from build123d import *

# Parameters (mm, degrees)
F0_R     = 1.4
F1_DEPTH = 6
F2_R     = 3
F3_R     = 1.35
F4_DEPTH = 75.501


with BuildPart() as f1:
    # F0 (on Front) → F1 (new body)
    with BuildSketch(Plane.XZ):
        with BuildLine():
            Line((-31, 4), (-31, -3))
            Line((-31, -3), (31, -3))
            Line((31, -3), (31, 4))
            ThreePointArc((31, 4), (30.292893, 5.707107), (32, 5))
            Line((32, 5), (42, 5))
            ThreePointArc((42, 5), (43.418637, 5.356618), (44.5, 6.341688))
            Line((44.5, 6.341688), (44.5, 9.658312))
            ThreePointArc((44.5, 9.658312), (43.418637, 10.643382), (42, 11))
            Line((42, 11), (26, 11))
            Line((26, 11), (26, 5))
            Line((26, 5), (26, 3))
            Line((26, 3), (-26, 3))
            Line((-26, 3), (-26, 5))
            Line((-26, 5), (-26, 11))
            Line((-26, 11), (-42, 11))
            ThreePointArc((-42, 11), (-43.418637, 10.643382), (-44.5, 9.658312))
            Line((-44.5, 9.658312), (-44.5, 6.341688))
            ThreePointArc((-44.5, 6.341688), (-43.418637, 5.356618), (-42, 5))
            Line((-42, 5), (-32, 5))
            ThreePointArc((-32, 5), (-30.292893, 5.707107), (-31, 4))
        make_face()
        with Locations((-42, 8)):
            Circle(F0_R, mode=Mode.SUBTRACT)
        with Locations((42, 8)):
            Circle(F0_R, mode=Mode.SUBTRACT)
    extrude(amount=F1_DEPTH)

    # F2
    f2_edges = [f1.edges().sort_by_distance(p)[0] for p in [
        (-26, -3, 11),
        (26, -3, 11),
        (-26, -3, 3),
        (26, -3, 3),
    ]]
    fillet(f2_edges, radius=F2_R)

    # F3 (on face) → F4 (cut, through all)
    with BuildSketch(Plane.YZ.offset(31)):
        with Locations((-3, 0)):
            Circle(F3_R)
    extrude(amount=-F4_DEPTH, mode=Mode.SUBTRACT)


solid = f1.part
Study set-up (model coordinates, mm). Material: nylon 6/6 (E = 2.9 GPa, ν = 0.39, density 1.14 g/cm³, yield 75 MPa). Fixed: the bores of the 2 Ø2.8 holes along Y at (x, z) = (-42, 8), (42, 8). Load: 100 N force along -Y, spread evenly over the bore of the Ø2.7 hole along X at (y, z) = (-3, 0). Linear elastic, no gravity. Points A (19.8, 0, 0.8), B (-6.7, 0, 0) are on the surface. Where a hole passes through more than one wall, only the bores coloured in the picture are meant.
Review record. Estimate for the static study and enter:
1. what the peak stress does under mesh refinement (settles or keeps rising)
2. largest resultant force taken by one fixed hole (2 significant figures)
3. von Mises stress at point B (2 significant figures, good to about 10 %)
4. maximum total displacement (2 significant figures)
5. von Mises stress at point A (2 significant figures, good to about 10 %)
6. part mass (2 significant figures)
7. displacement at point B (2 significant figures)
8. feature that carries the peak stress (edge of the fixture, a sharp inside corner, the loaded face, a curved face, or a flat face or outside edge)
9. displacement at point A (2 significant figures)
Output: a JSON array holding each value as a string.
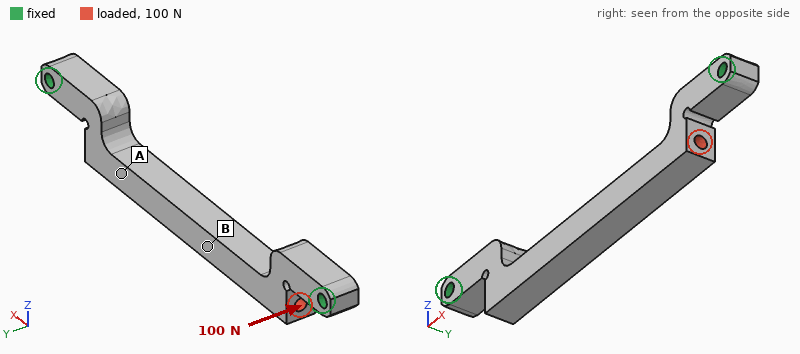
["keeps rising", "50 N", "13 MPa", "1.1 mm", "4.8 MPa", "3.7 g", "0.93 mm", "edge of the fixture", "0.66 mm"]
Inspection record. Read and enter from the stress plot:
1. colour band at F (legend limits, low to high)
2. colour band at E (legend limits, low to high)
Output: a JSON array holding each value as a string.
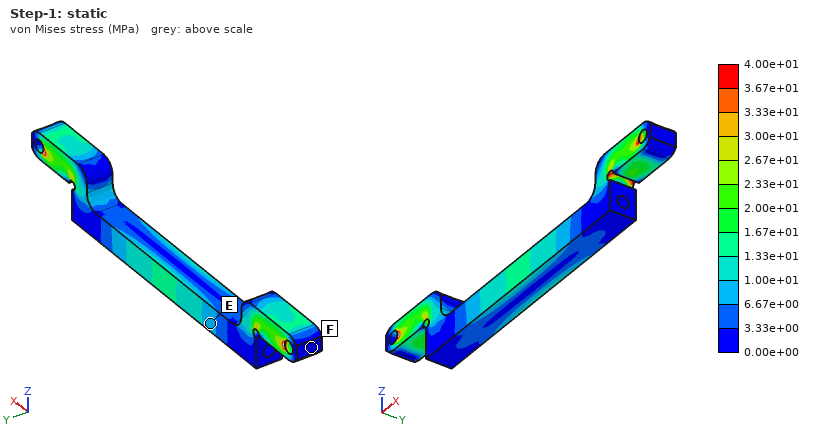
["0.00e+00 to 3.33e+00 MPa", "6.67e+00 to 1.00e+01 MPa"]
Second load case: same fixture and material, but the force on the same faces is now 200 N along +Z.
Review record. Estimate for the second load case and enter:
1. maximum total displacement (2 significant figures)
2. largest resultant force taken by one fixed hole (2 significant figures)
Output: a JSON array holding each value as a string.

["0.61 mm", "190 N"]
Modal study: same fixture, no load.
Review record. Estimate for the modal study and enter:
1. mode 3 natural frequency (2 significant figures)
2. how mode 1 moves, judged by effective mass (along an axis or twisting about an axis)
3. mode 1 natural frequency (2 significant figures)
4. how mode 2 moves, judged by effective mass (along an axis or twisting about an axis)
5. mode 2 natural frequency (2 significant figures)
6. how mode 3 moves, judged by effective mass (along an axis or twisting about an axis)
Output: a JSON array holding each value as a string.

["2800 Hz", "along Y", "1200 Hz", "along Z", "2200 Hz", "twisting about Z"]
